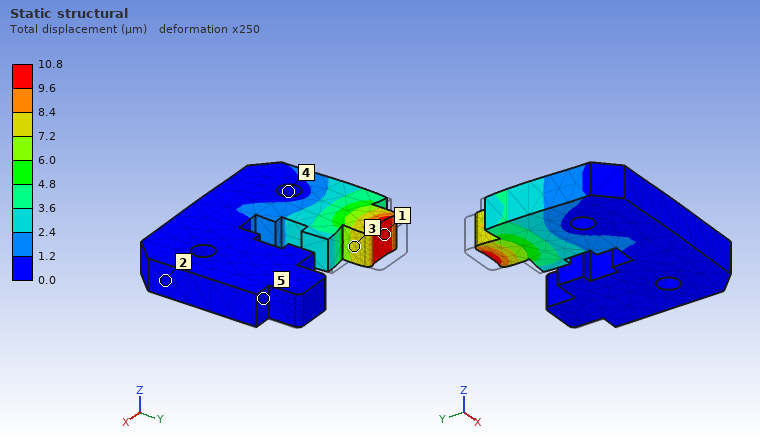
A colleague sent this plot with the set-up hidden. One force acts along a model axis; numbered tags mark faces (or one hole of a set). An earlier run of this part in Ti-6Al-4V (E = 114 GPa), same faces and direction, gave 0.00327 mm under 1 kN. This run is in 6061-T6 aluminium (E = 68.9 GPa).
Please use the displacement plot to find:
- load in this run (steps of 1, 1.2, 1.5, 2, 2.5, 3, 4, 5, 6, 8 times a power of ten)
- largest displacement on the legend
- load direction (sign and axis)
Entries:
2 kN
10.8 µm
-Y
